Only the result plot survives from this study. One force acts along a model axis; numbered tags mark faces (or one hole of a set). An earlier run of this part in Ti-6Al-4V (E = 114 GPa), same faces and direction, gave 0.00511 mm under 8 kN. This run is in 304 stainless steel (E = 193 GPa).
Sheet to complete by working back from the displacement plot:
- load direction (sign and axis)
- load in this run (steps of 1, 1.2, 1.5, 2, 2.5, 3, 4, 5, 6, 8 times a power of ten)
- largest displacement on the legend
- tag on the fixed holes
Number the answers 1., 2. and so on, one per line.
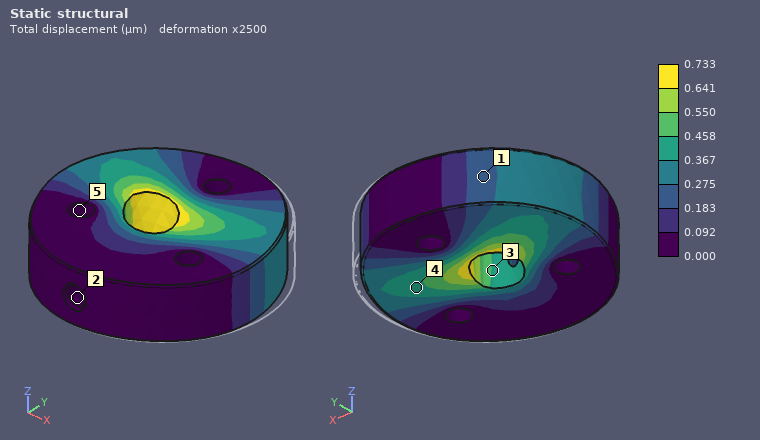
1. -X
2. 2 kN
3. 0.733 µm
4. 5
